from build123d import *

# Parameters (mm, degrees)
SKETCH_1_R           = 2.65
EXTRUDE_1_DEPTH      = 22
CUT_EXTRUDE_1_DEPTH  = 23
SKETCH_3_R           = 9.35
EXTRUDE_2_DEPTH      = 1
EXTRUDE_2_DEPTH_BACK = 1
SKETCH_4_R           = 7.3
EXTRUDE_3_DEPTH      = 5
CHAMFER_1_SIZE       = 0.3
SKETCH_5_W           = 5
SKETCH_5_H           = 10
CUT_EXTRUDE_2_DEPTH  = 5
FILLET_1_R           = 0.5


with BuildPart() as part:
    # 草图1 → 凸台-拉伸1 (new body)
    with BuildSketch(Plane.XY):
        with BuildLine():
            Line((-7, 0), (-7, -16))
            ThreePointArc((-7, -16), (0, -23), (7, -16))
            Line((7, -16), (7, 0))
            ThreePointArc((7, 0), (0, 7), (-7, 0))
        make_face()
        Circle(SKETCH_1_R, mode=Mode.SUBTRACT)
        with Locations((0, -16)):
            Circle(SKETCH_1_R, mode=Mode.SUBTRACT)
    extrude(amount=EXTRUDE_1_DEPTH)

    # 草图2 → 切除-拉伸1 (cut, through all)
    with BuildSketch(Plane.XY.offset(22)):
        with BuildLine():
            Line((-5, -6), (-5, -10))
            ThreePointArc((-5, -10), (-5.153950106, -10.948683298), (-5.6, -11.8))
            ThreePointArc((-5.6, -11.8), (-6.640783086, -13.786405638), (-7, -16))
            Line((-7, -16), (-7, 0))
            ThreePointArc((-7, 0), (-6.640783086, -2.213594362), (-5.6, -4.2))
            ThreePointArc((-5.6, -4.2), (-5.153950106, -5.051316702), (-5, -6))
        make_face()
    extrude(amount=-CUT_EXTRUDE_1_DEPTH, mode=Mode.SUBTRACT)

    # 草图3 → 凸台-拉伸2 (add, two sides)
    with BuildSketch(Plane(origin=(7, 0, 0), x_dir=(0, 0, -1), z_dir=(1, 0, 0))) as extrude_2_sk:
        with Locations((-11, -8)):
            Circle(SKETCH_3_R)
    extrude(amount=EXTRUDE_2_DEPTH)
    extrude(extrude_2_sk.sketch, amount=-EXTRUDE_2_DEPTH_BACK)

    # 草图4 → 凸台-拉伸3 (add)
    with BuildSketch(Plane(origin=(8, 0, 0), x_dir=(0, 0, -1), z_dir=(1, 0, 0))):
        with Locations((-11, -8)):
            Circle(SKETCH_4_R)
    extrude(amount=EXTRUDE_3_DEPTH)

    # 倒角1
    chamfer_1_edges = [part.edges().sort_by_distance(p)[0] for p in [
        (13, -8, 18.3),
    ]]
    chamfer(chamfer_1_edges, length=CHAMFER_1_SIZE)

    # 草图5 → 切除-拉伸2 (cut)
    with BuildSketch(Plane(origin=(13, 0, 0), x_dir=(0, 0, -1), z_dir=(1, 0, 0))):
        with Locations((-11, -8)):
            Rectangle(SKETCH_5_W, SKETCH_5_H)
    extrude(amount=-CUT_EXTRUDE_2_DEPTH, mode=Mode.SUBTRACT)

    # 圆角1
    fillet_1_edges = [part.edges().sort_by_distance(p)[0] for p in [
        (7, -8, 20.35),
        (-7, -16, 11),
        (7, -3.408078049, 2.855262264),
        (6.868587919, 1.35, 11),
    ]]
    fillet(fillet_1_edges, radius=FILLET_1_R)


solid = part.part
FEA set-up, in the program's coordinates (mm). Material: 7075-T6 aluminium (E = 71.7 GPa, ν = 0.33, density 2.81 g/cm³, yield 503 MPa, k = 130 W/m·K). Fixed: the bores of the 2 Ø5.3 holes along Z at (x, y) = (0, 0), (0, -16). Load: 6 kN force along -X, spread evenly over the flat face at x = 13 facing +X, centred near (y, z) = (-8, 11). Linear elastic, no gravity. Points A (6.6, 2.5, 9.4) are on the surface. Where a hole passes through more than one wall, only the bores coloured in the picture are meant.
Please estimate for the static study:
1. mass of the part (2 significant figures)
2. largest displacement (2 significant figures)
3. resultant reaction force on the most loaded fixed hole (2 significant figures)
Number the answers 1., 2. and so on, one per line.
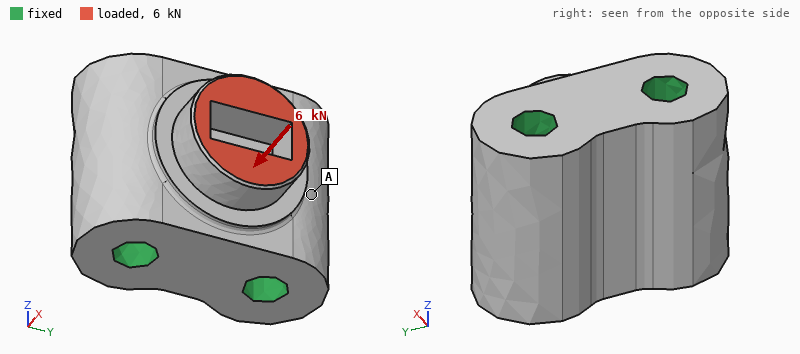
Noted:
1. 22 g
2. 6.8 µm
3. 3.3 kN
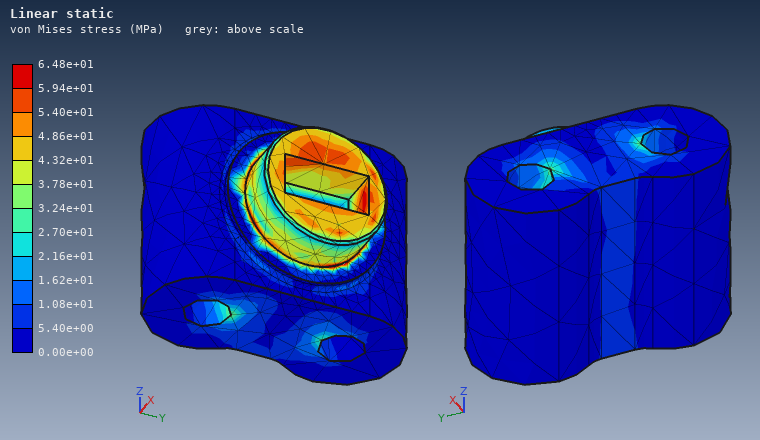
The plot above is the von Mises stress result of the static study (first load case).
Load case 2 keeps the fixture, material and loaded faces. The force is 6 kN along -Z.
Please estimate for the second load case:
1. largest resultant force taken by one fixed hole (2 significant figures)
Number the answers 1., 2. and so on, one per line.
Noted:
1. 3.0 kN
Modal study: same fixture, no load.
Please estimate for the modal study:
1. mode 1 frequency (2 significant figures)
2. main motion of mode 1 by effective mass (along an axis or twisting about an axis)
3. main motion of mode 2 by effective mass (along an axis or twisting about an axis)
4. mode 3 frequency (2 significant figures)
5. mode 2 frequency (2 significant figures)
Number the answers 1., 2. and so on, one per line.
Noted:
1. 67 kHz
2. along Z
3. along Y
4. 86 kHz
5. 82 kHz
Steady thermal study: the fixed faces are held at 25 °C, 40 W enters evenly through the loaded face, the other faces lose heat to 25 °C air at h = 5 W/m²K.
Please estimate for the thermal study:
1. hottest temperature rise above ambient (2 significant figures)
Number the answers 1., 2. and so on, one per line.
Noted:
1. 22 K
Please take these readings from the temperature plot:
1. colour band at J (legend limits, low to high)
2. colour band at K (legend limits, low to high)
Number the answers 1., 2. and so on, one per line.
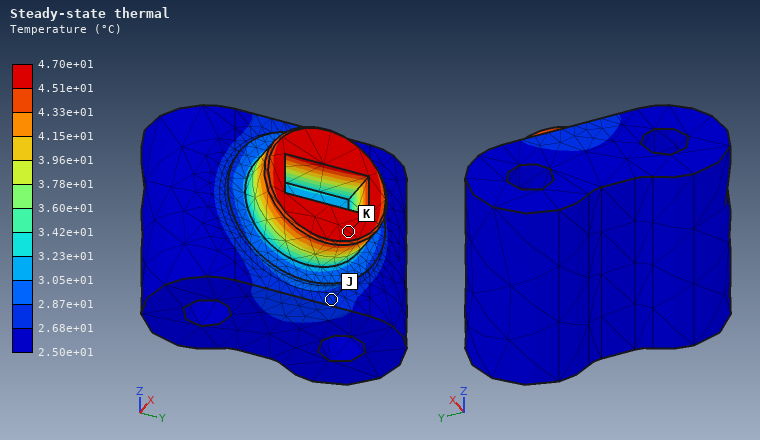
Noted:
1. 2.68e+01 to 2.87e+01 °C
2. 4.51e+01 to 4.70e+01 °C
